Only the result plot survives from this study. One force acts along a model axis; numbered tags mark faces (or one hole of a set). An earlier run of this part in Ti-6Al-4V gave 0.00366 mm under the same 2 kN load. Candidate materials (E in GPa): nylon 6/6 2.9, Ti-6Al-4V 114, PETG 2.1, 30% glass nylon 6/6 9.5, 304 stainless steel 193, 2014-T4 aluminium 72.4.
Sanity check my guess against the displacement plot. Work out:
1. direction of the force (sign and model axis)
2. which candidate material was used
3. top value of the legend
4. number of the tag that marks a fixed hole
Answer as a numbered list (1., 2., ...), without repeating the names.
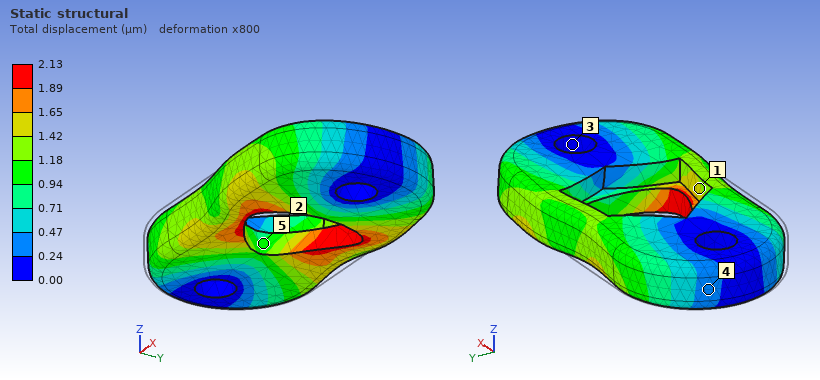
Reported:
1. +X
2. 304 stainless steel
3. 2.13 µm
4. 3
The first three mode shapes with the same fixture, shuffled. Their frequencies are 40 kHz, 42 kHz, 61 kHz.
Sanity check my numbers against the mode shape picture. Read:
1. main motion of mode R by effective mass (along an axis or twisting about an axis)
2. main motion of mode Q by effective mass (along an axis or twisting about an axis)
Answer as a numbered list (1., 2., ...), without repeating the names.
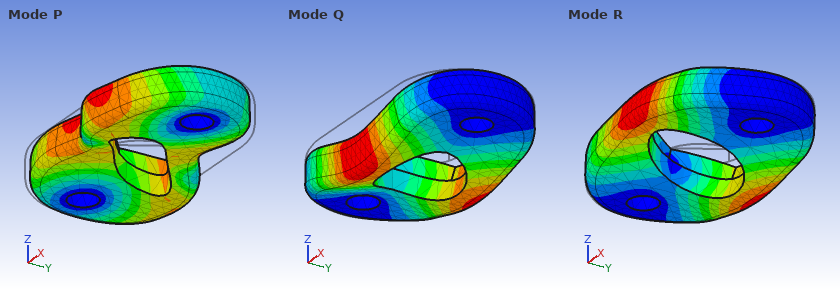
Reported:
1. twisting about X
2. along Z
